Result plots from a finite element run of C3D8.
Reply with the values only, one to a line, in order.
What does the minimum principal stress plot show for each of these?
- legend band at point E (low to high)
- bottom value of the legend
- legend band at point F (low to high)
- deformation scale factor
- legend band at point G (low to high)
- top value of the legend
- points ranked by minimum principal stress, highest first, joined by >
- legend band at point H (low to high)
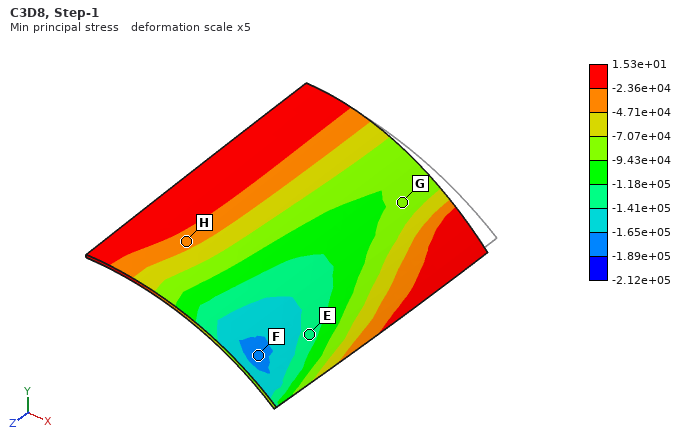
-1.41e+05 to -1.18e+05
-2.12e+05
-1.89e+05 to -1.65e+05
5
-9.43e+04 to -7.07e+04
1.53e+01
H > G > E > F
-4.71e+04 to -2.36e+04
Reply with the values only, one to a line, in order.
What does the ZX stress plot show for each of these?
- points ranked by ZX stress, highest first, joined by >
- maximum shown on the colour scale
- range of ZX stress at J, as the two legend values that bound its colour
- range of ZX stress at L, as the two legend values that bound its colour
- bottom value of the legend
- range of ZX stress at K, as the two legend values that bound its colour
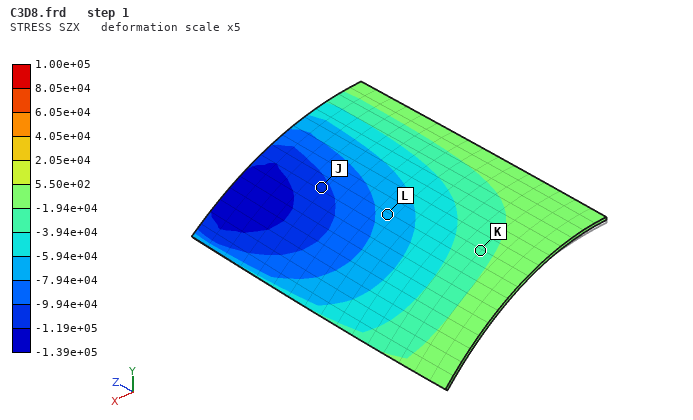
K > L > J
1.00e+05
-1.19e+05 to -9.94e+04
-7.94e+04 to -5.94e+04
-1.39e+05
-3.94e+04 to -1.94e+04
